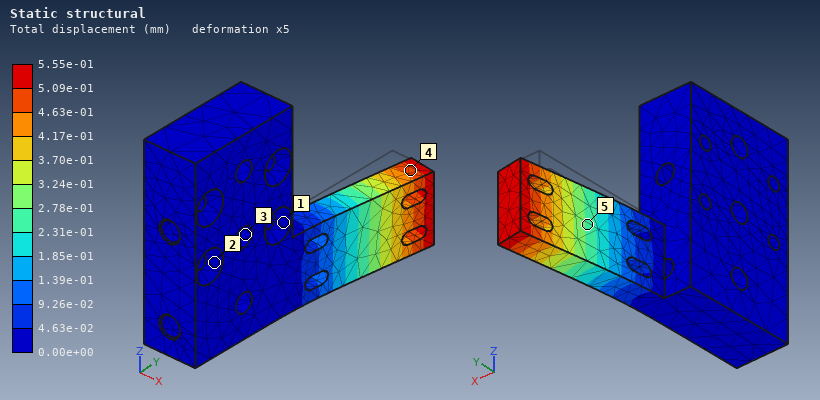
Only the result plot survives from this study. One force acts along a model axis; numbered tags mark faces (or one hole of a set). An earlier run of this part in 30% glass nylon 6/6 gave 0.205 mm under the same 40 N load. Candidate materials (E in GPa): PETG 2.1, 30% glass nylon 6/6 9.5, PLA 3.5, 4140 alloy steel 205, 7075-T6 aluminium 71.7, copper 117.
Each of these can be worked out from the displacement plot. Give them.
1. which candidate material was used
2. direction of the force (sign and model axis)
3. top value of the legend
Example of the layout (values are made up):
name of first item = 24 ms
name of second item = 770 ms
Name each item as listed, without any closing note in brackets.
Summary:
which candidate material was used = PLA
direction of the force = +X
top value of the legend = 5.55e-01 mm
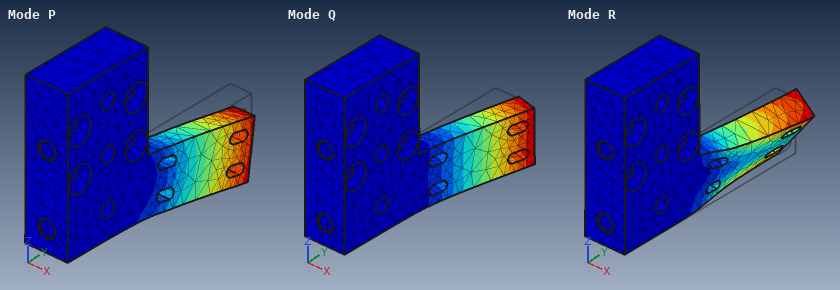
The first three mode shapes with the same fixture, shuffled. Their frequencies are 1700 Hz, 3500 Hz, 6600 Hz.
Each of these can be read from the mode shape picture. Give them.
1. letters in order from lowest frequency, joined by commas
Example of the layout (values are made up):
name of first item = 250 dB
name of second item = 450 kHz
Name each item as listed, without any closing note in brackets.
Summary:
letters in order from lowest frequency, joined by commas = Q, P, R
